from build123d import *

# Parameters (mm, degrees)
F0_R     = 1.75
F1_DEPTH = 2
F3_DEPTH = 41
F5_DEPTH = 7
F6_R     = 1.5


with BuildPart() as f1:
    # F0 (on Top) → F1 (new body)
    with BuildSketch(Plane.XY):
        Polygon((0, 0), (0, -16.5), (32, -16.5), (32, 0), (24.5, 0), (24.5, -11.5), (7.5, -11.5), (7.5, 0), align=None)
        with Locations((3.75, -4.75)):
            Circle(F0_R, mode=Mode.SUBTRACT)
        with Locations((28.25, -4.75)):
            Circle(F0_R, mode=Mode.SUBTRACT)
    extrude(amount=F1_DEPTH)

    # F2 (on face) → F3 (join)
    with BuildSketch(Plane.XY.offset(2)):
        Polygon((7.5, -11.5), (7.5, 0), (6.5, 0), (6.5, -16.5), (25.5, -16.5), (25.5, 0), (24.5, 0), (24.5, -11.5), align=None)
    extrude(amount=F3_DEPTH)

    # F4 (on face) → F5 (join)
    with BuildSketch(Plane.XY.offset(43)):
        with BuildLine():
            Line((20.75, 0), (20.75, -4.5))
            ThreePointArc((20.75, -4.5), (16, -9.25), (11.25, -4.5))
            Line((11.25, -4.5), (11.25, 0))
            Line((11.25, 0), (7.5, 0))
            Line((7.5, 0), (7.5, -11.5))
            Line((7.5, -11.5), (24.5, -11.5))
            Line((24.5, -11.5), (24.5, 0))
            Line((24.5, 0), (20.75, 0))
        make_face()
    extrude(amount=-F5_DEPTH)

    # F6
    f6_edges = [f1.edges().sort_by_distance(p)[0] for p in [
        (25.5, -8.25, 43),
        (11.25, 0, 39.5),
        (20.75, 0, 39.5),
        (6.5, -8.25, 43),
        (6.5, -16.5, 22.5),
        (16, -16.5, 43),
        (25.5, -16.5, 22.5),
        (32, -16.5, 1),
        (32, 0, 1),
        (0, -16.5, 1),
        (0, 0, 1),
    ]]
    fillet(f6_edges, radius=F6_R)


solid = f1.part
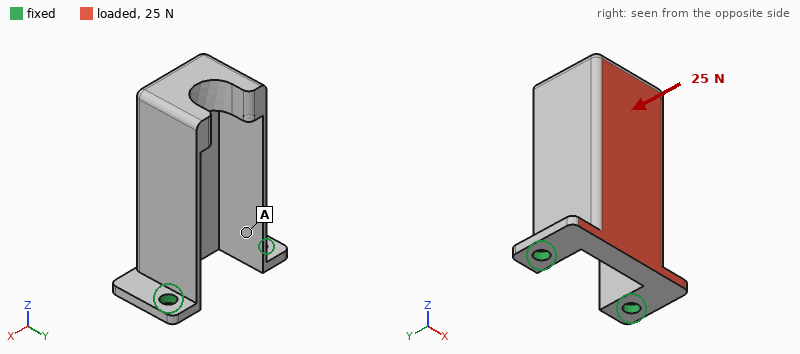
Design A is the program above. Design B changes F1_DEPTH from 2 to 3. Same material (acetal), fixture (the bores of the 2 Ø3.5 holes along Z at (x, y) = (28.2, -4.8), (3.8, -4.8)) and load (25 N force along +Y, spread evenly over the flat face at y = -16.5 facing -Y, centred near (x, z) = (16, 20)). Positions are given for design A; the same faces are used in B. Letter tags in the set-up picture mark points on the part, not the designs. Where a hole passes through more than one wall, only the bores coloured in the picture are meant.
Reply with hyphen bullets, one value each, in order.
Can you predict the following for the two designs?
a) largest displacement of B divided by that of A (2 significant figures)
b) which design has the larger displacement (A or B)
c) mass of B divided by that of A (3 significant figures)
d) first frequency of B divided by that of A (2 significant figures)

- 0.47
- A
- 1.03
- 1.4
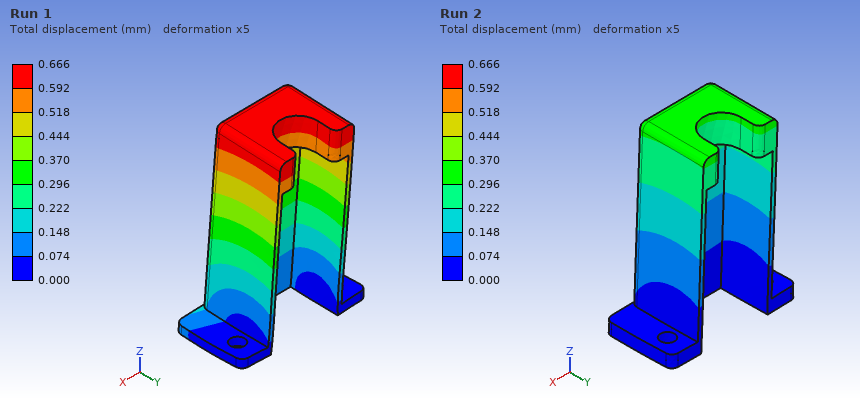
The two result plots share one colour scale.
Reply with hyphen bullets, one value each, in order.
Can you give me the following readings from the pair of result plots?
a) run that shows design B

- Run 2
